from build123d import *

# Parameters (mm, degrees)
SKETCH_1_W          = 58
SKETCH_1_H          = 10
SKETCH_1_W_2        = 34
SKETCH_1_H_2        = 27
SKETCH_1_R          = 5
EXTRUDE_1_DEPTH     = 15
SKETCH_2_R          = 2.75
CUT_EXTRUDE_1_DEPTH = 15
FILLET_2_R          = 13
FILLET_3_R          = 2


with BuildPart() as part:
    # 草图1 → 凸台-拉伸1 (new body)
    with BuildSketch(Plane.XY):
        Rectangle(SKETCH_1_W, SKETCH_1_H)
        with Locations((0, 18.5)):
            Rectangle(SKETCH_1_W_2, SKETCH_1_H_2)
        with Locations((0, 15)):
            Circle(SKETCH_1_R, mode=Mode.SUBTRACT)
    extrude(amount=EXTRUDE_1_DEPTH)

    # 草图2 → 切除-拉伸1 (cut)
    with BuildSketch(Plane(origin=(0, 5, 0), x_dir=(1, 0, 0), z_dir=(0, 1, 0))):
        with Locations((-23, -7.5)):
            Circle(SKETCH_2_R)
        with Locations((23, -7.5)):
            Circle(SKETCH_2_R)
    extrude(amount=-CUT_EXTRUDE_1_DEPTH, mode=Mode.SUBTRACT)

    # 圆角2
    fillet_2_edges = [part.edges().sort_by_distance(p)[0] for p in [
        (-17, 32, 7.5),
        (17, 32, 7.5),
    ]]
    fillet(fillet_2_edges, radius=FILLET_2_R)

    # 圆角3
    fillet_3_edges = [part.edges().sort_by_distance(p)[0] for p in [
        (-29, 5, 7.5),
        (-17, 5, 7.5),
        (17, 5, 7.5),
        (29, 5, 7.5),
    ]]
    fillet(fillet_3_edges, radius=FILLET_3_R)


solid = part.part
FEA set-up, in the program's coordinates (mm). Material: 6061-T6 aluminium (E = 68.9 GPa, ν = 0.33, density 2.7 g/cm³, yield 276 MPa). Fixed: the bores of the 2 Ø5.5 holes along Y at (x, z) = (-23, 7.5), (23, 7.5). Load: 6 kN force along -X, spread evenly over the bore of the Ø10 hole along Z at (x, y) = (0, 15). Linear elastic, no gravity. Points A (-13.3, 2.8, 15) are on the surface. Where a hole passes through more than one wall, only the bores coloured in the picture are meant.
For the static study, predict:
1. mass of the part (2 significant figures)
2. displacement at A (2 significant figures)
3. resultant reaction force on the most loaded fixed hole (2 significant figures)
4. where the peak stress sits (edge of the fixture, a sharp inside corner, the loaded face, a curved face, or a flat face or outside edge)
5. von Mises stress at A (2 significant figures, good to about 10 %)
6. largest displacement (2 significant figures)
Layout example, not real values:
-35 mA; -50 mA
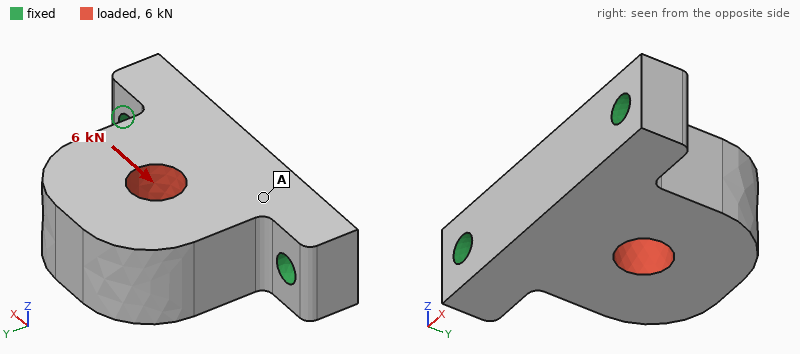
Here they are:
53 g; 4.3 µm; 3.7 kN; a curved face; 14 MPa; 21 µm
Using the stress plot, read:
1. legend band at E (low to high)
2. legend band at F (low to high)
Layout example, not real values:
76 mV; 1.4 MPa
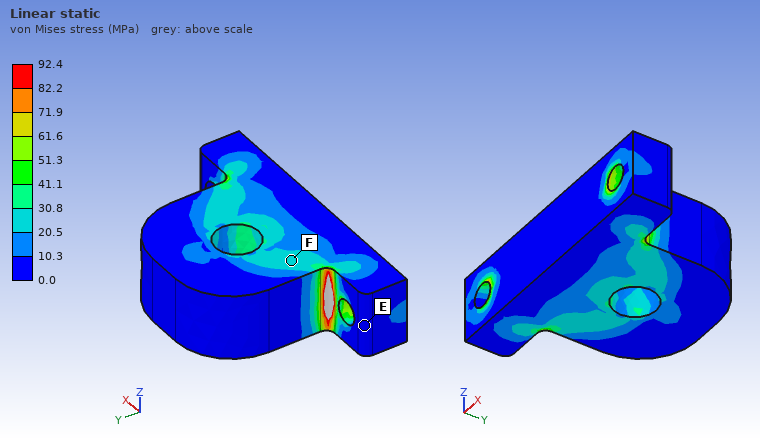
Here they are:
0.0 to 10.3 MPa; 20.5 to 30.8 MPa
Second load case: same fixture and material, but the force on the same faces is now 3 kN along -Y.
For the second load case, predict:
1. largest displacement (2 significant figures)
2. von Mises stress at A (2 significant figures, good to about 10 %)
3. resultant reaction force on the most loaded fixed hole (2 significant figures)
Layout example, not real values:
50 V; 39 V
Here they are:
7.3 µm; 7.3 MPa; 1.6 kN
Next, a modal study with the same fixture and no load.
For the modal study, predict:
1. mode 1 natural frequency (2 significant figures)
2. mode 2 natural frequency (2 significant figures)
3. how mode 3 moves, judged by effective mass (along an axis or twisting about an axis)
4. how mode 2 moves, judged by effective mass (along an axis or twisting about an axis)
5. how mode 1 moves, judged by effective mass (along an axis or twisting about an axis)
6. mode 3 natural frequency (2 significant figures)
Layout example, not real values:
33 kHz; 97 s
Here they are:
5600 Hz; 15 kHz; along Y; along X; along Z; 17 kHz
